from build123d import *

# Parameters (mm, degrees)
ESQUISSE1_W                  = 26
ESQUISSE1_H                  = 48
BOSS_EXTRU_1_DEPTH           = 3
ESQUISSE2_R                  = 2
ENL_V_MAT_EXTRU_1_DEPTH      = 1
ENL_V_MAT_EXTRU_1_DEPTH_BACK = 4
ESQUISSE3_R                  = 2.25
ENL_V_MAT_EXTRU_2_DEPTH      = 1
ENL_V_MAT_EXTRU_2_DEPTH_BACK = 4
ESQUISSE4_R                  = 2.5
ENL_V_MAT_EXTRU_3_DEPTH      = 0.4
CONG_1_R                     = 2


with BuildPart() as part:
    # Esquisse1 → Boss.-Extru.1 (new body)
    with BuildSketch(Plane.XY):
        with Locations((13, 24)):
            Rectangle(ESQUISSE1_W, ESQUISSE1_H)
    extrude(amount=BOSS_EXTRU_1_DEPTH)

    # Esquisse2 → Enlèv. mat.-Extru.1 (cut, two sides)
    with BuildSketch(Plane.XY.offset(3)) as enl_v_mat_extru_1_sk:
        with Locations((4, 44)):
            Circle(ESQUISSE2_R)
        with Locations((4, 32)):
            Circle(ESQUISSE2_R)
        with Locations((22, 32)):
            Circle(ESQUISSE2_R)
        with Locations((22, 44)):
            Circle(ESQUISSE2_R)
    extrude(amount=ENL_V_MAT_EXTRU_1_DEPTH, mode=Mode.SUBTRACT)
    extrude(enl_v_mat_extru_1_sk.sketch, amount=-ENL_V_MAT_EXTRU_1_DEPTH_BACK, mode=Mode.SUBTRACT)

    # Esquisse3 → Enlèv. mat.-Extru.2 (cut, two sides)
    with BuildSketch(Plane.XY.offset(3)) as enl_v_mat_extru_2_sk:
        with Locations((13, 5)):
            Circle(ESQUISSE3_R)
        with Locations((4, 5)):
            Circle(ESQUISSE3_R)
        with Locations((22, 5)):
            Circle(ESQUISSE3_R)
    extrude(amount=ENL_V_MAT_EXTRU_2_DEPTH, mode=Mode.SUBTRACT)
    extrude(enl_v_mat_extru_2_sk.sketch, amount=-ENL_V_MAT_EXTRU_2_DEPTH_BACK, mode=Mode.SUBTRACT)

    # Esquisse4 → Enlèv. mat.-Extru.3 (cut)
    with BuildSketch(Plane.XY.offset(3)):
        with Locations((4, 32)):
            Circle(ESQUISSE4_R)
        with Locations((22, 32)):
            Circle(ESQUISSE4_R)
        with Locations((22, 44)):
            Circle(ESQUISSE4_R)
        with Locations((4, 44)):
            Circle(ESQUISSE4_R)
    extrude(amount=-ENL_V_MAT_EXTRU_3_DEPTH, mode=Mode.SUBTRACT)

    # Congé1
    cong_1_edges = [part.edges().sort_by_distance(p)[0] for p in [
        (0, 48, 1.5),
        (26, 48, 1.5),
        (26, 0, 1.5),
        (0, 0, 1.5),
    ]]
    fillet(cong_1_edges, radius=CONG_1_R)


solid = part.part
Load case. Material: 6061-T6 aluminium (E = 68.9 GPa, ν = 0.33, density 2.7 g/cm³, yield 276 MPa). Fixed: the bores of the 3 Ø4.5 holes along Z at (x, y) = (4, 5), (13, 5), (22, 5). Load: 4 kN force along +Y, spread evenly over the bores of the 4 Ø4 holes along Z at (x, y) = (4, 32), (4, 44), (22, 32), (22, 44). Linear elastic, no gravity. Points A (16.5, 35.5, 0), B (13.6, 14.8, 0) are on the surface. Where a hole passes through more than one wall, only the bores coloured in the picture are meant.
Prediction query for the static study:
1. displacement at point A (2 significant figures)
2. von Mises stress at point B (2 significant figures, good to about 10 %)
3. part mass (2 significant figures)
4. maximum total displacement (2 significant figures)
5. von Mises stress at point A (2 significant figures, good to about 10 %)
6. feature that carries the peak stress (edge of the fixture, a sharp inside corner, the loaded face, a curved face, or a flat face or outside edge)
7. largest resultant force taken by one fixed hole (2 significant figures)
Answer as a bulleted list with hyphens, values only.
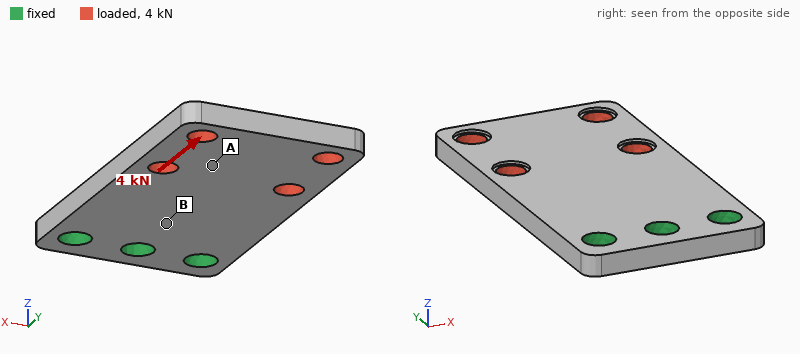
- 0.086 mm
- 69 MPa
- 9.3 g
- 0.16 mm
- 49 MPa
- the loaded face
- 1.4 kN
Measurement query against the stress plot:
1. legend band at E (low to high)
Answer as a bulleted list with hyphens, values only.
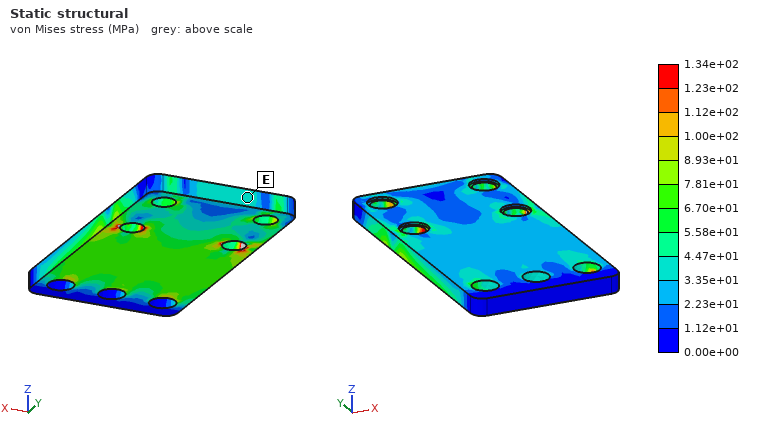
- 3.35e+01 to 4.47e+01 MPa
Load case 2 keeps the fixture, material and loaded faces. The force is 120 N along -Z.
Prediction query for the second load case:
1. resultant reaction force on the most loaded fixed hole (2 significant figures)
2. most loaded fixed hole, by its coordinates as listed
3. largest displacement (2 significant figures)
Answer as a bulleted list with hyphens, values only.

- 86 N
- (13, 5)
- 0.45 mm
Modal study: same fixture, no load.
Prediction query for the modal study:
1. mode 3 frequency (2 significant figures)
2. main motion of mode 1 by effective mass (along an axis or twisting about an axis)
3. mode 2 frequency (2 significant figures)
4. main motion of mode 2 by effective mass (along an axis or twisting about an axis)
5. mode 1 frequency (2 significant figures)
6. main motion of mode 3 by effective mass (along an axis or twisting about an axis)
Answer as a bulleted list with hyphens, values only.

- 8700 Hz
- along Z
- 5100 Hz
- twisting about Y
- 1500 Hz
- along Z
